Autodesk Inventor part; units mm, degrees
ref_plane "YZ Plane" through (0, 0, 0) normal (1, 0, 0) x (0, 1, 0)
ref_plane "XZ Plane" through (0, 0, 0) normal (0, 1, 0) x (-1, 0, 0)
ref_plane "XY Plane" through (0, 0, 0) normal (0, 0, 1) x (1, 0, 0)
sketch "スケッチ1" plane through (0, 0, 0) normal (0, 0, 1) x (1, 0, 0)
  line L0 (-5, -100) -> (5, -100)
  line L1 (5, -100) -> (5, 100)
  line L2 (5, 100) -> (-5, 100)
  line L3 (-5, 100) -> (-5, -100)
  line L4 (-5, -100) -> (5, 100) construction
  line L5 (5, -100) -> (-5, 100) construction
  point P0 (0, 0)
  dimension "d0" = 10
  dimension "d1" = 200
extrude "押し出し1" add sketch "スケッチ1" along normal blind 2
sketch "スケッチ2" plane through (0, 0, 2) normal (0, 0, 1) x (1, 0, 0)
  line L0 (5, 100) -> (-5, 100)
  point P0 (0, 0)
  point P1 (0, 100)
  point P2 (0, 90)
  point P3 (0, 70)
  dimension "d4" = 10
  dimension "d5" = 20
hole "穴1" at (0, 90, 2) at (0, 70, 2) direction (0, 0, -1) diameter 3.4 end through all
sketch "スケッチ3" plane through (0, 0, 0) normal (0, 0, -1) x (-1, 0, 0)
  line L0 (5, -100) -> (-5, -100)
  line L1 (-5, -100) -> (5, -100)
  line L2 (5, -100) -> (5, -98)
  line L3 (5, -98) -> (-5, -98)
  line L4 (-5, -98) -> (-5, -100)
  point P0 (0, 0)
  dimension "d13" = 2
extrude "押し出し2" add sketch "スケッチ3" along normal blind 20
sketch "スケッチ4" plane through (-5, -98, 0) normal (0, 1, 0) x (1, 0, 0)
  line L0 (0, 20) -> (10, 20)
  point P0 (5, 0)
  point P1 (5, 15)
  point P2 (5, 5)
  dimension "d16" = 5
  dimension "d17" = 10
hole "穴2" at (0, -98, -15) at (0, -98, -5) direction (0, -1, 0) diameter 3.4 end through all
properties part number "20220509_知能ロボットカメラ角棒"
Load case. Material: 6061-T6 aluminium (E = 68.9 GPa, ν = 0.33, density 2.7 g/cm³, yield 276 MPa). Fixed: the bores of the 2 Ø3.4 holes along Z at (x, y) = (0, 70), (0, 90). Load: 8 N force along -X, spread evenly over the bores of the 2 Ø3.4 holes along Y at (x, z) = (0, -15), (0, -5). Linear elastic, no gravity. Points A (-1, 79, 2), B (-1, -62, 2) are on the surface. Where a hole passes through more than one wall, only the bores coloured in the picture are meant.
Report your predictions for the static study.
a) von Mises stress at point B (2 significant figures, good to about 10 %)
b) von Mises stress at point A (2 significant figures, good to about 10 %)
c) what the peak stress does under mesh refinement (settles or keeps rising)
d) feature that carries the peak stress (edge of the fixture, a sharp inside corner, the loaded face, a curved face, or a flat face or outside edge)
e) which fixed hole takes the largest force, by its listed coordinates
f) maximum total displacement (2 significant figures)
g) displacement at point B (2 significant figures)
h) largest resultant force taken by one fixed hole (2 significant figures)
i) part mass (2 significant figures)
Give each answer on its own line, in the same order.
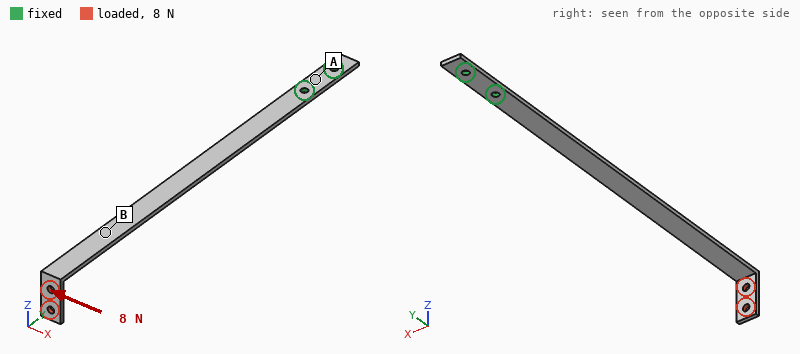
12 MPa
4.0 MPa
keeps rising
edge of the fixture
(0, 70)
1.7 mm
0.78 mm
38 N
12 g
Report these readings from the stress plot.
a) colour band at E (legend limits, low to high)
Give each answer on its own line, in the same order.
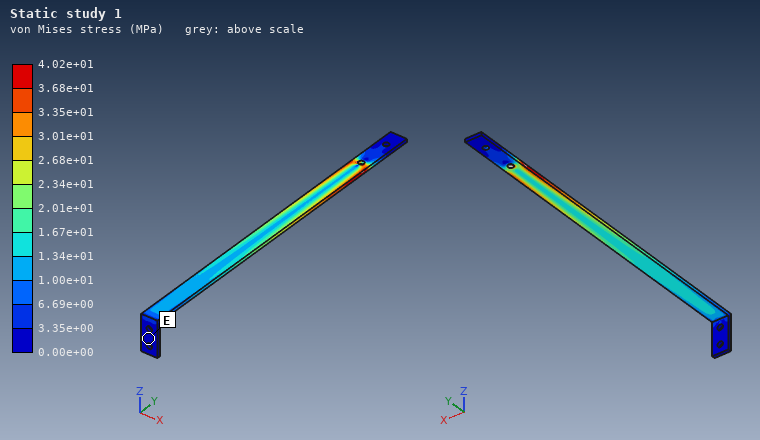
0.00e+00 to 3.35e+00 MPa
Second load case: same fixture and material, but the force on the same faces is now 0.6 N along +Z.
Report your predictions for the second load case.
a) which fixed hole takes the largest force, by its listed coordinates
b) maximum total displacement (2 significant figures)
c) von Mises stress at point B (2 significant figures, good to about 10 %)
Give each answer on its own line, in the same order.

(0, 70)
2.1 mm
3.4 MPa
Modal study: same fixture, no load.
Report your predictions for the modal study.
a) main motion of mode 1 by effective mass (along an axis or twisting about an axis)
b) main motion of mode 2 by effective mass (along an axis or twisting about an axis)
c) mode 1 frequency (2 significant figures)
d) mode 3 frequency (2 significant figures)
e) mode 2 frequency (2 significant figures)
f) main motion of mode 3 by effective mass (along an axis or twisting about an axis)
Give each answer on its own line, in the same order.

along Z
along X
48 Hz
310 Hz
230 Hz
along Z
